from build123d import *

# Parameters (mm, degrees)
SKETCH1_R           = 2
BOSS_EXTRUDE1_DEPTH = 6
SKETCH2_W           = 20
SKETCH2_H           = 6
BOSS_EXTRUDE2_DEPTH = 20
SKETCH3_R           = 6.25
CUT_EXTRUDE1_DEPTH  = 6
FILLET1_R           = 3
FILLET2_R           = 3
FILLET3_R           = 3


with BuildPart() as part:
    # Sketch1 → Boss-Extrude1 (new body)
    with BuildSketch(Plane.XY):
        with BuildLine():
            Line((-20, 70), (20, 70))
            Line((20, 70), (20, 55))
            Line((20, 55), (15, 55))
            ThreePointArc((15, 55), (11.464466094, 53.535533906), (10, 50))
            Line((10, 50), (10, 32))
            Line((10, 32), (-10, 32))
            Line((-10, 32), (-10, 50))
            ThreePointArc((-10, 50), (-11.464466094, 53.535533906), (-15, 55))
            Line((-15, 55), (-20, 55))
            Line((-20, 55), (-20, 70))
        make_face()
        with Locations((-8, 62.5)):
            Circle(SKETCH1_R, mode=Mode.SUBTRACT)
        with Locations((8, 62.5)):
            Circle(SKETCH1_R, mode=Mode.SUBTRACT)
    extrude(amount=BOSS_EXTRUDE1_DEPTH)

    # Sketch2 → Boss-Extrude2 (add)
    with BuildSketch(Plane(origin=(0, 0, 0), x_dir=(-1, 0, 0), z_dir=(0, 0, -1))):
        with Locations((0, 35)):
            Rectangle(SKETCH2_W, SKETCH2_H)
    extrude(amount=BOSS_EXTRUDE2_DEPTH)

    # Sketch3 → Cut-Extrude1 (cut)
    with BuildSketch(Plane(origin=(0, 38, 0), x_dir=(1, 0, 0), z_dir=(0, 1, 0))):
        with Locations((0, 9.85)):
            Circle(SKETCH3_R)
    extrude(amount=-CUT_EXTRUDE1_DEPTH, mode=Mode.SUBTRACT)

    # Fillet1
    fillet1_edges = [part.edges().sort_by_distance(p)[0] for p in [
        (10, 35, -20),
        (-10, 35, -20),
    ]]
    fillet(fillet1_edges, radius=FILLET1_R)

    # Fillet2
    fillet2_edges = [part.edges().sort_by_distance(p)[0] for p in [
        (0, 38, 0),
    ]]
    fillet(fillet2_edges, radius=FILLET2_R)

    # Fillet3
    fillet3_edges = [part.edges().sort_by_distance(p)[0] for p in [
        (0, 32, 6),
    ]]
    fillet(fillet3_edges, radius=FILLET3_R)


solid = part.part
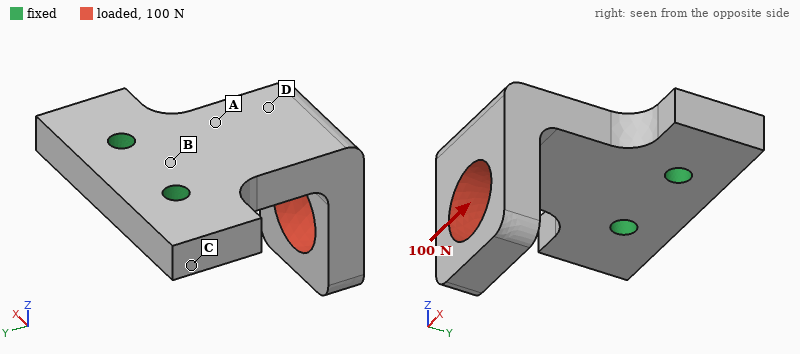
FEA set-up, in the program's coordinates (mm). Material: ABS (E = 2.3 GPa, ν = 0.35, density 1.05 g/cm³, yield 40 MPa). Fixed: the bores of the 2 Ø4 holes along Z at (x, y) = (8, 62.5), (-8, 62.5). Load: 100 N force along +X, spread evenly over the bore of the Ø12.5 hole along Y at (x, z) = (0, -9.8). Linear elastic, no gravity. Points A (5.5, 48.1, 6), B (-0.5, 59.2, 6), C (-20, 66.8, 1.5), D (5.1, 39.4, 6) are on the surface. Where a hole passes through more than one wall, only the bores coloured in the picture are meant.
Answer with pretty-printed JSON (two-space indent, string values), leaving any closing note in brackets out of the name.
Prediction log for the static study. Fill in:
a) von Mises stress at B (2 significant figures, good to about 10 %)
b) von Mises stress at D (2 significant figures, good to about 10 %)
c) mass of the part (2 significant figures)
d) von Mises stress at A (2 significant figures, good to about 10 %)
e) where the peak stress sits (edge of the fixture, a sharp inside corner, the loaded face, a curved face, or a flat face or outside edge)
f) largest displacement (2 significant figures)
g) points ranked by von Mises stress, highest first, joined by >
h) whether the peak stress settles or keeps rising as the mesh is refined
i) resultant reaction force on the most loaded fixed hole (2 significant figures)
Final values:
{
  "von Mises stress at B": "3.0 MPa",
  "von Mises stress at D": "5.5 MPa",
  "mass of the part": "8.3 g",
  "von Mises stress at A": "7.5 MPa",
  "where the peak stress sits": "edge of the fixture",
  "largest displacement": "0.65 mm",
  "points ranked by von Mises stress, highest first, joined by >": "A > D > B > C",
  "whether the peak stress settles or keeps rising as the mesh is refined": "keeps rising",
  "resultant reaction force on the most loaded fixed hole": "170 N"
}
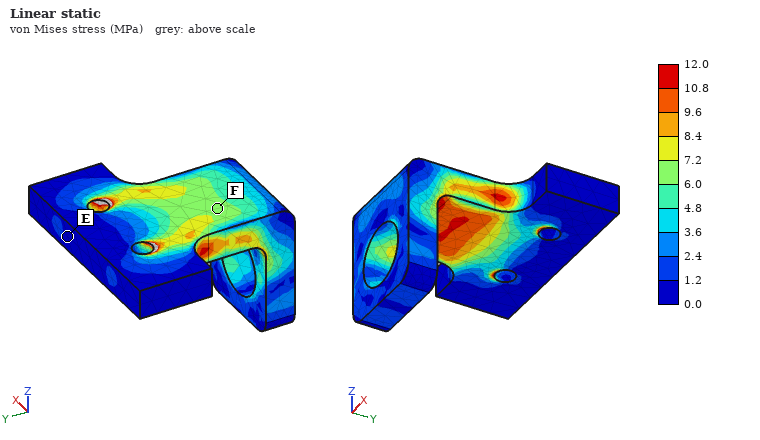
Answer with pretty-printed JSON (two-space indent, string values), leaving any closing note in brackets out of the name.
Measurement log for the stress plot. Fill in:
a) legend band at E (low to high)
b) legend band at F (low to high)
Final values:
{
  "legend band at E": "0.0 to 1.2 MPa",
  "legend band at F": "6.0 to 7.2 MPa"
}
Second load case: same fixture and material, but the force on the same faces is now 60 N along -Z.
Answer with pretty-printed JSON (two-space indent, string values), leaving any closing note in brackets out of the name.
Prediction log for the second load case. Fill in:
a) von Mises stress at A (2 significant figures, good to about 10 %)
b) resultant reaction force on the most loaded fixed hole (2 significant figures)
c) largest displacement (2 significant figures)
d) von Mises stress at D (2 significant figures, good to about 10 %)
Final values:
{
  "von Mises stress at A": "6.3 MPa",
  "resultant reaction force on the most loaded fixed hole": "30 N",
  "largest displacement": "0.72 mm",
  "von Mises stress at D": "2.1 MPa"
}
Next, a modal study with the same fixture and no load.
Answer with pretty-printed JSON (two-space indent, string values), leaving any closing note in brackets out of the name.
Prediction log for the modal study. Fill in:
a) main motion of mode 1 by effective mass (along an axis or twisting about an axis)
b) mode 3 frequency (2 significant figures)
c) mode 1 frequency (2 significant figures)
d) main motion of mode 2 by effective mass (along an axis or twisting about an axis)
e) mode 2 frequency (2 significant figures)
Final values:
{
  "main motion of mode 1 by effective mass": "along Z",
  "mode 3 frequency": "2500 Hz",
  "mode 1 frequency": "930 Hz",
  "main motion of mode 2 by effective mass": "along X",
  "mode 2 frequency": "1600 Hz"
}
